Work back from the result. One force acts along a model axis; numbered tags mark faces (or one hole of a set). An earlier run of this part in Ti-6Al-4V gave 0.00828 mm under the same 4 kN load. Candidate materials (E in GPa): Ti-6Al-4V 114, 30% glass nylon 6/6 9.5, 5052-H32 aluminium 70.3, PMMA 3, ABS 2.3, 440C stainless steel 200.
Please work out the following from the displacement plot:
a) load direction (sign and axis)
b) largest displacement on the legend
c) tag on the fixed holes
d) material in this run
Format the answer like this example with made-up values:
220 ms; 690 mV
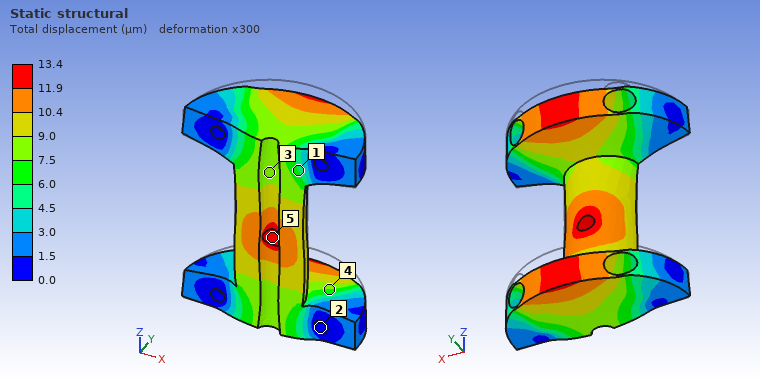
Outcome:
-Z; 13.4 µm; 2; 5052-H32 aluminium
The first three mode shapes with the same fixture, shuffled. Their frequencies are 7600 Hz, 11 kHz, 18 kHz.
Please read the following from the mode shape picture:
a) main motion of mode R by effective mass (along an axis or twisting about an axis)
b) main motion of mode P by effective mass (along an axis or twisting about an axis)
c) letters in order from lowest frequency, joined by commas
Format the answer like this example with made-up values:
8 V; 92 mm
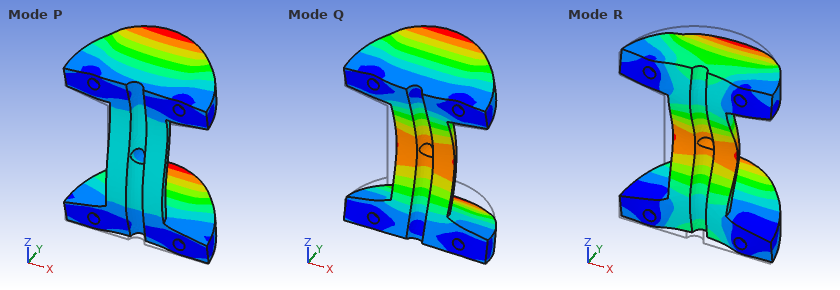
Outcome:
along Y; along Z; Q, P, R
